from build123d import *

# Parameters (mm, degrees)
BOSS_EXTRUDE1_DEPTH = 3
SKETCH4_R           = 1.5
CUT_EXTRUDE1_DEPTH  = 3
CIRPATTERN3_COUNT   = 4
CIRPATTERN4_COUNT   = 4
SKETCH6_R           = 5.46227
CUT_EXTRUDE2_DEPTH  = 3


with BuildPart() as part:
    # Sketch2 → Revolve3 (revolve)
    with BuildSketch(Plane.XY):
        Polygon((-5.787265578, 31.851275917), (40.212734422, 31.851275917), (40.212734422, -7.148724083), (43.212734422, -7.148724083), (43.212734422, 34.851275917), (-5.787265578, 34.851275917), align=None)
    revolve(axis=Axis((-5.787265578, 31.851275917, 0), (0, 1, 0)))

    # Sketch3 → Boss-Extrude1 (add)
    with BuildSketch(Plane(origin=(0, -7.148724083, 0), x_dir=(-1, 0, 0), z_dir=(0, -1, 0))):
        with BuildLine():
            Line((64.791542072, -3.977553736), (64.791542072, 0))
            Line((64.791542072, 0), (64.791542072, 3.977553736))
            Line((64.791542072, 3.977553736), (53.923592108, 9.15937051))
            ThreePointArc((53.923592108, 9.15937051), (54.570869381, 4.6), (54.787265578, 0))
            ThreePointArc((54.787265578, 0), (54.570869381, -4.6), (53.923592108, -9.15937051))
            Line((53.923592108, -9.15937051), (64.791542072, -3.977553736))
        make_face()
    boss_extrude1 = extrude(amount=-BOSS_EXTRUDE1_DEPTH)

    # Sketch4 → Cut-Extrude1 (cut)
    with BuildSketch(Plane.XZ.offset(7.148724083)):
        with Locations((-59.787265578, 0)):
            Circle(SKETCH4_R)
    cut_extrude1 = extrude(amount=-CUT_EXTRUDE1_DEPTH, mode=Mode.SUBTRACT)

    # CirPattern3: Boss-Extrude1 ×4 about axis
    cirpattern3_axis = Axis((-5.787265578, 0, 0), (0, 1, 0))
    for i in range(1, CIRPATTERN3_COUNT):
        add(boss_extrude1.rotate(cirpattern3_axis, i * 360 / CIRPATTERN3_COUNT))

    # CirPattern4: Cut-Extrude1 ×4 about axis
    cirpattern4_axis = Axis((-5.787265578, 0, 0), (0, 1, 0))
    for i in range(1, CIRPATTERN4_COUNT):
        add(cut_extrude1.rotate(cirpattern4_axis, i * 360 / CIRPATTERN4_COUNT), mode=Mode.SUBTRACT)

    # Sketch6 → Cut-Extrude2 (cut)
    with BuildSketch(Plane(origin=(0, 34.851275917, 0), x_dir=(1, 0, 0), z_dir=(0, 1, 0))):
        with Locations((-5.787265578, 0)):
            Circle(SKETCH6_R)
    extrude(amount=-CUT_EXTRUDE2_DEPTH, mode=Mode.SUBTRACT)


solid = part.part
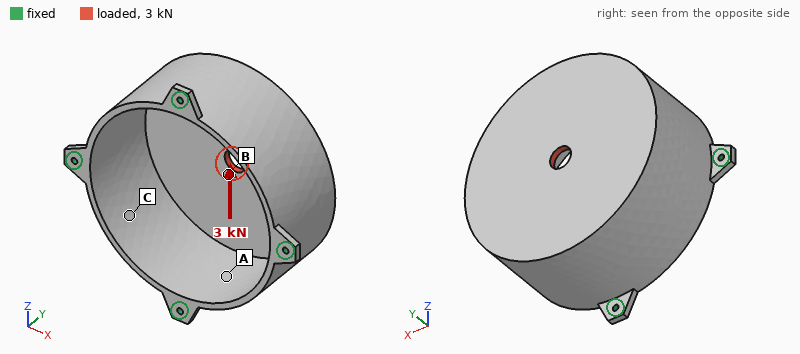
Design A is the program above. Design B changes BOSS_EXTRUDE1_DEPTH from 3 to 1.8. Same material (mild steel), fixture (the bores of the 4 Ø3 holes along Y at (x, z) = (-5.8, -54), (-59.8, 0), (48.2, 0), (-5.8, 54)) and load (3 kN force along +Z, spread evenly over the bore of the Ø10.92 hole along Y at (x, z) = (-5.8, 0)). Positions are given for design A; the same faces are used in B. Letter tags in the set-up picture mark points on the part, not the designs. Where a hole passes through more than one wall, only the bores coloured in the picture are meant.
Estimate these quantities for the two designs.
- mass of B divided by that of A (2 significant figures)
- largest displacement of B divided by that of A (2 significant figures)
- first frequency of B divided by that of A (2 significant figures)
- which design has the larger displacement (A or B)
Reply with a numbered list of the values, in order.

1. 0.99
2. 1.7
3. 0.91
4. B
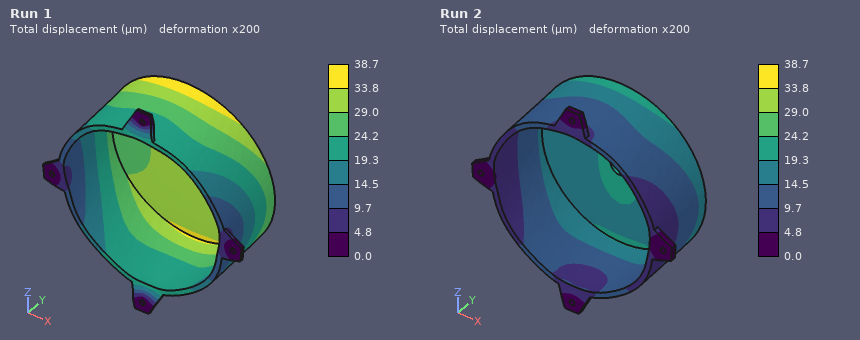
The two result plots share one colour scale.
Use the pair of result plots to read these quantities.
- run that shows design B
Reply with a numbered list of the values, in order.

1. Run 1
